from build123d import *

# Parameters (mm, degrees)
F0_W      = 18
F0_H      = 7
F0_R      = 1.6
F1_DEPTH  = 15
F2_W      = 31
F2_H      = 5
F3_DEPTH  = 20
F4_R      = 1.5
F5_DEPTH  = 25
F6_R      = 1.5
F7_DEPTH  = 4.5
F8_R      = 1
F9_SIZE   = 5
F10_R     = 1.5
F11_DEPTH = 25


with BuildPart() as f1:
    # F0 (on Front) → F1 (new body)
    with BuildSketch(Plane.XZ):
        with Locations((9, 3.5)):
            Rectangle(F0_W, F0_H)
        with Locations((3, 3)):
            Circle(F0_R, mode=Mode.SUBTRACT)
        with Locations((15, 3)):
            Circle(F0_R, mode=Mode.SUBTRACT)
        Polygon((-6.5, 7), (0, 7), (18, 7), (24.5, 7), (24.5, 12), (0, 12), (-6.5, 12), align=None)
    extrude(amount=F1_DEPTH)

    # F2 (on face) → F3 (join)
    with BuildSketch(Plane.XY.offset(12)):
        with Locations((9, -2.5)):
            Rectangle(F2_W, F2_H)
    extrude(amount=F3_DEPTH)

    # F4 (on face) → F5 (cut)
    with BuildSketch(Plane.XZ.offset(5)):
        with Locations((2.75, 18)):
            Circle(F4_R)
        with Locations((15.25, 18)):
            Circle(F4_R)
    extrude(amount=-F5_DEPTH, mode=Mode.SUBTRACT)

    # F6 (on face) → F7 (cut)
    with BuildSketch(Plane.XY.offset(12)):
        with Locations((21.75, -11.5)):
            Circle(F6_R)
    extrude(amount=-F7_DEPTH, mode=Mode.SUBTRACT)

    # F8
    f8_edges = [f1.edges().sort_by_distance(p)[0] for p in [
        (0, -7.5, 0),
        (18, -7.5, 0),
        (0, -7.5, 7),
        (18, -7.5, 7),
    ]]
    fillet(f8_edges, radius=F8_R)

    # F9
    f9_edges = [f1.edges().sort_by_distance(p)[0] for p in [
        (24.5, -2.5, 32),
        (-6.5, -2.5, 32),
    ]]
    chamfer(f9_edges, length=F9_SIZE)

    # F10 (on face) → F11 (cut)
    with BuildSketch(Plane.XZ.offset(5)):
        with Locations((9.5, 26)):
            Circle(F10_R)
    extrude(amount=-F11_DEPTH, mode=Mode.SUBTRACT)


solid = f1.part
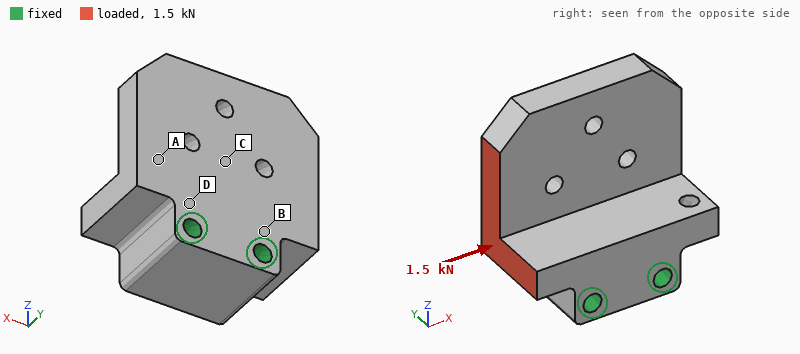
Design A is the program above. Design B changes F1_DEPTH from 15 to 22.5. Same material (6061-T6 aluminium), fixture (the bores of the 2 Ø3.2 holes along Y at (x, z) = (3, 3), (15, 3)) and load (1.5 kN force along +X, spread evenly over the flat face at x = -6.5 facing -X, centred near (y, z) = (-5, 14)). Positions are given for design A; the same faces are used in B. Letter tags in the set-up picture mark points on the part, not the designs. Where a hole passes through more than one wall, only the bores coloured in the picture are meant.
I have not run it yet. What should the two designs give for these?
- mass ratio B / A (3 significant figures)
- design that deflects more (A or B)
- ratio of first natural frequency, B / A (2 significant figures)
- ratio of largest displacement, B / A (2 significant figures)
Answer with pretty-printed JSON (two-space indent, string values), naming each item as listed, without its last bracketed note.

{
  "mass ratio B / A": "1.29",
  "design that deflects more": "A",
  "ratio of first natural frequency, B / A": "1.0",
  "ratio of largest displacement, B / A": "0.78"
}
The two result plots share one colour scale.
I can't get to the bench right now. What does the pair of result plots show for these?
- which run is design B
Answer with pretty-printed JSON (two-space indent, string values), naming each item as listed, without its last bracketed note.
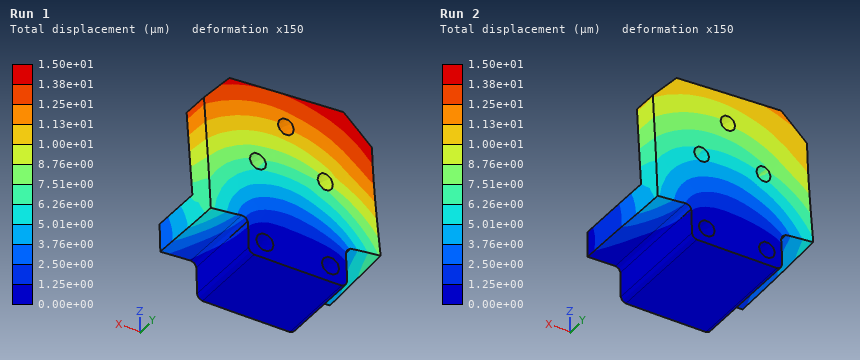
{
  "which run is design B": "Run 2"
}
